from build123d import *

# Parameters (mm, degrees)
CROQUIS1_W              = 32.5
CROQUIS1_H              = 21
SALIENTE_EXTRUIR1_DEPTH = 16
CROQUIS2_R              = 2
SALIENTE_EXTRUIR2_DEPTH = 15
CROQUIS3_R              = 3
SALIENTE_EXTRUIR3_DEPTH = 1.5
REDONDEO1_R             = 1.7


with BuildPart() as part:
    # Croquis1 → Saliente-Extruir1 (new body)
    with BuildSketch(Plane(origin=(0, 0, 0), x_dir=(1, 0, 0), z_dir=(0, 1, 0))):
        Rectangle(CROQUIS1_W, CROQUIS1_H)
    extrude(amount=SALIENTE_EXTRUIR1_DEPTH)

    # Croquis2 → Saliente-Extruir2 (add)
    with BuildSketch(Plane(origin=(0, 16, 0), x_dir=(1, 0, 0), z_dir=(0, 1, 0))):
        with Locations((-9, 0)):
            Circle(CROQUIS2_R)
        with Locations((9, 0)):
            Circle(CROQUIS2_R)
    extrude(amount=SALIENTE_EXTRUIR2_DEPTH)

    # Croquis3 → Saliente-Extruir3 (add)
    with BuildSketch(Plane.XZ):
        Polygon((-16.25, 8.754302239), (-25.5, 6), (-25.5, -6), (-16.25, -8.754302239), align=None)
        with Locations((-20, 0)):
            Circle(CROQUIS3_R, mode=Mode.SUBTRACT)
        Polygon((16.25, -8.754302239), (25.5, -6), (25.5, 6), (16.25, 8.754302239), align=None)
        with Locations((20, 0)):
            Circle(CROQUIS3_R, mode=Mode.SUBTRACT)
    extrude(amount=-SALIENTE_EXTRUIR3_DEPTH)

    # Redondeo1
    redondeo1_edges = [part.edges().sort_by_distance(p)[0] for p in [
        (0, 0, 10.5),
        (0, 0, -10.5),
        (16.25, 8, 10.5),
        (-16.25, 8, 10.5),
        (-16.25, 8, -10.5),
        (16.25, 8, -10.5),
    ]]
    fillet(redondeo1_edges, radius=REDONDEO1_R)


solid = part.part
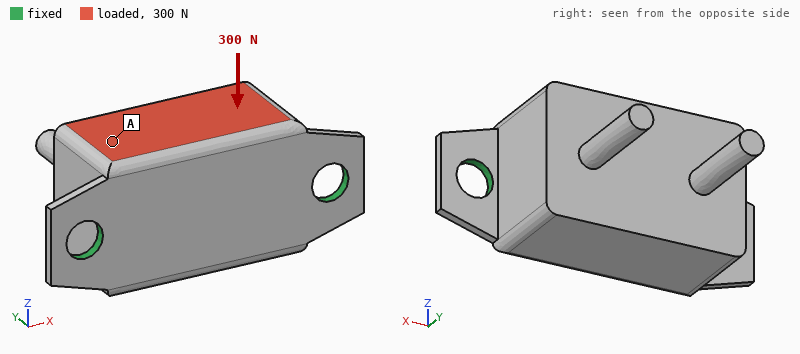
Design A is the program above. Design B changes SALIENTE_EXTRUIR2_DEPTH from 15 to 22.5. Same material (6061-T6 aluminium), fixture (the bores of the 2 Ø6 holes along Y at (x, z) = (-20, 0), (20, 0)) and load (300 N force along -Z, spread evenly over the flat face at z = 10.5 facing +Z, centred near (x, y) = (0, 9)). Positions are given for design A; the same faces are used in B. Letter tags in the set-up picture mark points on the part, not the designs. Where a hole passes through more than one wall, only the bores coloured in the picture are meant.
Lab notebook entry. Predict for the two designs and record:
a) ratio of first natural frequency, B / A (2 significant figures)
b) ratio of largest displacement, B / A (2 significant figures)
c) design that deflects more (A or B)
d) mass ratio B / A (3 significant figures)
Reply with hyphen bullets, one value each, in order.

- 0.91
- 1.2
- B
- 1.02
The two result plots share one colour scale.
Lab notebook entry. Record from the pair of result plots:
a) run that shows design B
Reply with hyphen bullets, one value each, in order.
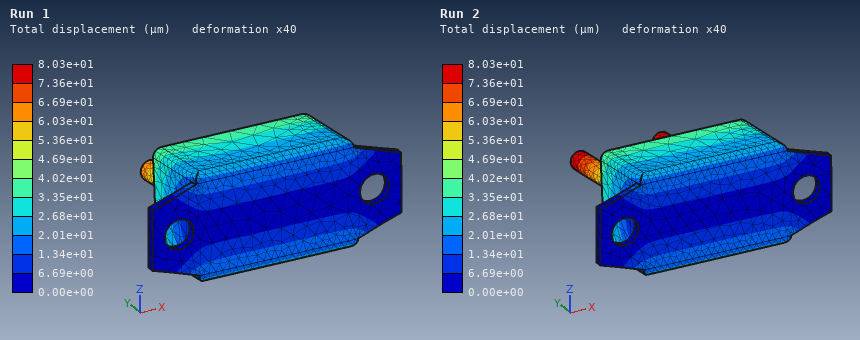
- Run 2
